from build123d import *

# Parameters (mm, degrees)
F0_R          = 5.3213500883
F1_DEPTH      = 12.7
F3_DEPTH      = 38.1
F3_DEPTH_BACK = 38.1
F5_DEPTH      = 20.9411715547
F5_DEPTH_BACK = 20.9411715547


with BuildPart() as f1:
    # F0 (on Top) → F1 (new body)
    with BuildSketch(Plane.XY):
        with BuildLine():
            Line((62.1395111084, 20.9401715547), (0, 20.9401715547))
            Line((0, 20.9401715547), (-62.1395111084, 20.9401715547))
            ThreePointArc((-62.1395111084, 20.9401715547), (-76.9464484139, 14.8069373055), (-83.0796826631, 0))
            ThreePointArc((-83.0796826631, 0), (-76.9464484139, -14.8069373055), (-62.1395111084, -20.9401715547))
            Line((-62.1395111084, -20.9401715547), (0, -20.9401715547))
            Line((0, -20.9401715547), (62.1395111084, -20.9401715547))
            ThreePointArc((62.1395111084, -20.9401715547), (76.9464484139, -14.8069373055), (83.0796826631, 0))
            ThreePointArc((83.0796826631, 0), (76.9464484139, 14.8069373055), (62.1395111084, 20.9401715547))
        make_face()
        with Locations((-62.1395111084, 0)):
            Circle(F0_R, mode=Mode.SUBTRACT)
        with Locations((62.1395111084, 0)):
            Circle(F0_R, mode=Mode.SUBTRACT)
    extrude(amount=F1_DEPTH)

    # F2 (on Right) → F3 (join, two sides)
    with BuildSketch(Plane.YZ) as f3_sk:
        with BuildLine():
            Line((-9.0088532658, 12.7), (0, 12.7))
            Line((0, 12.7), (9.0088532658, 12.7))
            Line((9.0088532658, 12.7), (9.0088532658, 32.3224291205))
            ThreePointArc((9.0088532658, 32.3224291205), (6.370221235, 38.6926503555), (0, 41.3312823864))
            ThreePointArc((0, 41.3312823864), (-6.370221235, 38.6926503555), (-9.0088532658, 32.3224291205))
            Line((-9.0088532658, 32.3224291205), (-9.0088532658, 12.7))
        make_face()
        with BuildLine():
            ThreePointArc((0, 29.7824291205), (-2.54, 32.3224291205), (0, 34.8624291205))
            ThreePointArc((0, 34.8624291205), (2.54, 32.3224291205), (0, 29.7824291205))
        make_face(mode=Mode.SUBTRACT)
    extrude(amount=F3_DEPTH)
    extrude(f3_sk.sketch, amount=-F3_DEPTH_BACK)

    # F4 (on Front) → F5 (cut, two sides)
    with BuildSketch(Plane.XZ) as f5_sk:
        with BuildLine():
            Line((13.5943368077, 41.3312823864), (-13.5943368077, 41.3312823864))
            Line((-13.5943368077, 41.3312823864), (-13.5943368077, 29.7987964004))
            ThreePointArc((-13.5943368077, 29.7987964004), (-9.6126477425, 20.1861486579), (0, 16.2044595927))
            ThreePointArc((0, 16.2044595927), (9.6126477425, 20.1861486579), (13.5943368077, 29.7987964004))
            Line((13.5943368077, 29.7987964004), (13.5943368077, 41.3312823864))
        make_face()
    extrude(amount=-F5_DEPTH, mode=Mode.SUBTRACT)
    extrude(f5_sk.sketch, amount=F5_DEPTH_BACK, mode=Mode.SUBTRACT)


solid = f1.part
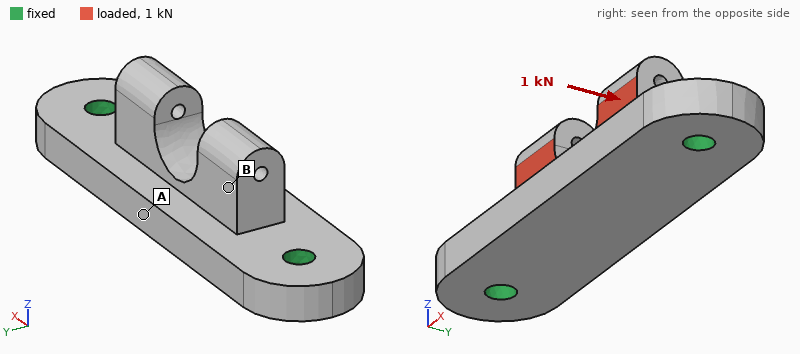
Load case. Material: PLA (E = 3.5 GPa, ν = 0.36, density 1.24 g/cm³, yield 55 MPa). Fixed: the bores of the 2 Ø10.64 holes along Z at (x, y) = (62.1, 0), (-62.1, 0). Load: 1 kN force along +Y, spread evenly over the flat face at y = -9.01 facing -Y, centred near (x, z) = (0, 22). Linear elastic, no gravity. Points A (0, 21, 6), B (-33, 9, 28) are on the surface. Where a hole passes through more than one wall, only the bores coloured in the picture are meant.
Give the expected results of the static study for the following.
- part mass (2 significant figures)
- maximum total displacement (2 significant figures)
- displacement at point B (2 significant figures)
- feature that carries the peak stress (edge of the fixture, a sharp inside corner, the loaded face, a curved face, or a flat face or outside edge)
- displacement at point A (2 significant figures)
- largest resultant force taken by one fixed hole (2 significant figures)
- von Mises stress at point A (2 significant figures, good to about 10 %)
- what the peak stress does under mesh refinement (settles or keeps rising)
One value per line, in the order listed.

130 g
0.34 mm
0.22 mm
edge of the fixture
0.17 mm
500 N
3.0 MPa
keeps rising
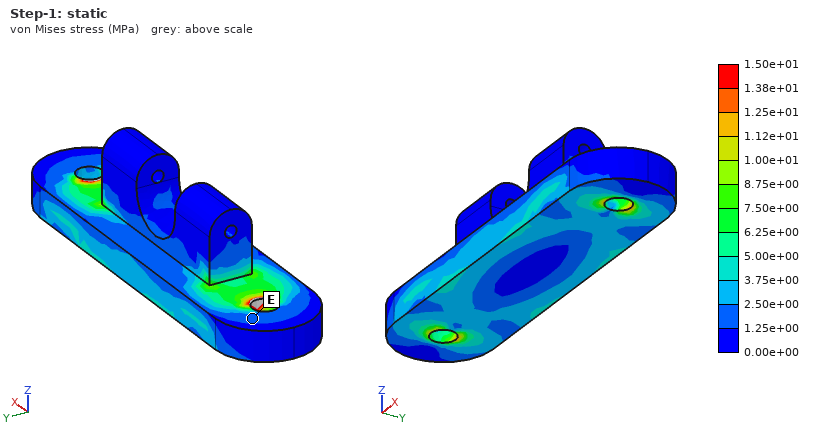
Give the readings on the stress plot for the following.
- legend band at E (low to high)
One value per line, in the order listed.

1.25e+00 to 2.50e+00 MPa
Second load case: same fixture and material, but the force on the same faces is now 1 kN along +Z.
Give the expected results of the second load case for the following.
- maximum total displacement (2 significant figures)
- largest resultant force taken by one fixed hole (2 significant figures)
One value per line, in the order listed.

0.30 mm
540 N
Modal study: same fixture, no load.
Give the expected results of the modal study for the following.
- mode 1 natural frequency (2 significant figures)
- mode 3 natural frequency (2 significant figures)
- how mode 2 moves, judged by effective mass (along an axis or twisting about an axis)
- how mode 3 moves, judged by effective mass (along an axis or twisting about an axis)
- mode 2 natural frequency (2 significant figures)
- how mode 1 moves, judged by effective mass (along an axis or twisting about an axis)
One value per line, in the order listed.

1300 Hz
2300 Hz
along Y
along Y
1400 Hz
along Z
